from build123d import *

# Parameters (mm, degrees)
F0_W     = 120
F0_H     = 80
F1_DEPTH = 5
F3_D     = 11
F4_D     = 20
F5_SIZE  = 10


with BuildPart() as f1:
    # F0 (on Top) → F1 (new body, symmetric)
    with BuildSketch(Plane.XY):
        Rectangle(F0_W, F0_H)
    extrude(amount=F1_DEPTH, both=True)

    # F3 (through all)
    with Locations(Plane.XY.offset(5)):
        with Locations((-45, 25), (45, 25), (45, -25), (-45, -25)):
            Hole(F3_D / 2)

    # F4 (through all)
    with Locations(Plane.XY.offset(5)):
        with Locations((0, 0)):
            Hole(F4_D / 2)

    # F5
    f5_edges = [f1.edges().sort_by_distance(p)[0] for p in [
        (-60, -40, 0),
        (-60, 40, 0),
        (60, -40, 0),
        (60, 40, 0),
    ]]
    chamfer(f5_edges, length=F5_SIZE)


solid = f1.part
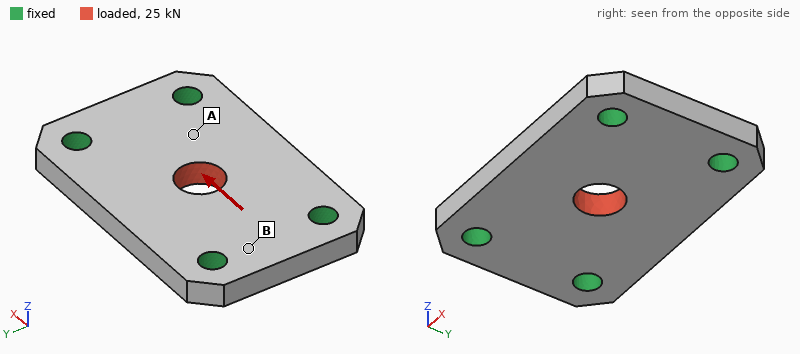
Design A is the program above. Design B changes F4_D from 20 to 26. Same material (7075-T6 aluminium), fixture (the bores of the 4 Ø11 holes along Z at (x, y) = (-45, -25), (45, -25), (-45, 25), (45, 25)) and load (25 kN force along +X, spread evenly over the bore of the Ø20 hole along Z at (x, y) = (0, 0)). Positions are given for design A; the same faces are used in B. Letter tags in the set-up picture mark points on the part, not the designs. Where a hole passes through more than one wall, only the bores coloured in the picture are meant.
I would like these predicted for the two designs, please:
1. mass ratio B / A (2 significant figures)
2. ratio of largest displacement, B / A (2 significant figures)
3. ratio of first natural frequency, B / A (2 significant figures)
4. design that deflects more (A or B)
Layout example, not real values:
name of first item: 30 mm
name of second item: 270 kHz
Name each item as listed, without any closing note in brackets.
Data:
mass ratio B / A: 0.98
ratio of largest displacement, B / A: 0.86
ratio of first natural frequency, B / A: 1.0
design that deflects more: A
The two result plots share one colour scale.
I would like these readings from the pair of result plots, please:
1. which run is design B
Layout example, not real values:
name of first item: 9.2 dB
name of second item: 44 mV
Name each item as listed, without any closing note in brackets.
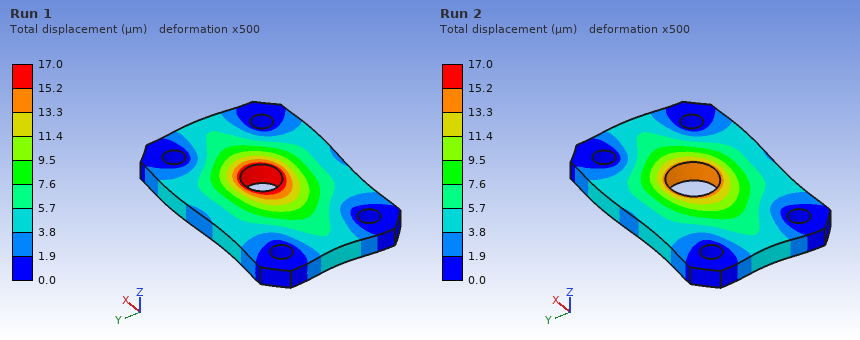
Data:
which run is design B: Run 2
